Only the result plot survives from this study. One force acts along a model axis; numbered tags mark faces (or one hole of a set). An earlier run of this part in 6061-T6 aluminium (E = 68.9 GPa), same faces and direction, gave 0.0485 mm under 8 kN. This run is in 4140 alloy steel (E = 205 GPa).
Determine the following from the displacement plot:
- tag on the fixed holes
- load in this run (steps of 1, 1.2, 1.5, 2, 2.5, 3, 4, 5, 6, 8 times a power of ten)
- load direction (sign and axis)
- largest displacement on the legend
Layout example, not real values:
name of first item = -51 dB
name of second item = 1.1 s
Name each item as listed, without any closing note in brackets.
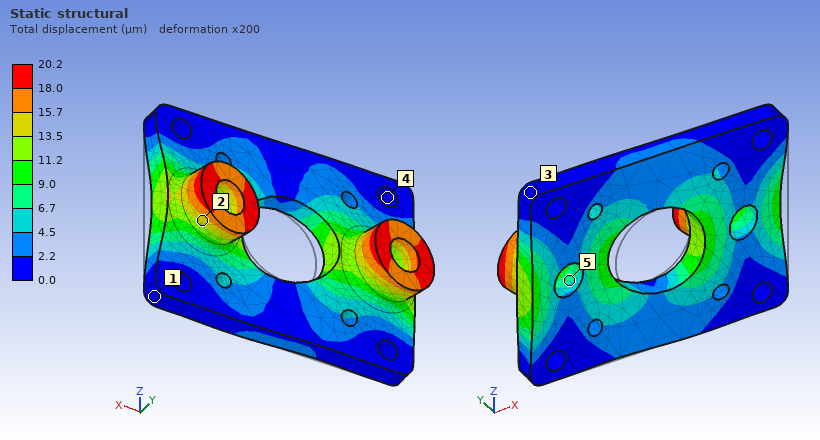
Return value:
tag on the fixed holes = 4
load in this run = 10 kN
load direction = -X
largest displacement on the legend = 20.2 µm
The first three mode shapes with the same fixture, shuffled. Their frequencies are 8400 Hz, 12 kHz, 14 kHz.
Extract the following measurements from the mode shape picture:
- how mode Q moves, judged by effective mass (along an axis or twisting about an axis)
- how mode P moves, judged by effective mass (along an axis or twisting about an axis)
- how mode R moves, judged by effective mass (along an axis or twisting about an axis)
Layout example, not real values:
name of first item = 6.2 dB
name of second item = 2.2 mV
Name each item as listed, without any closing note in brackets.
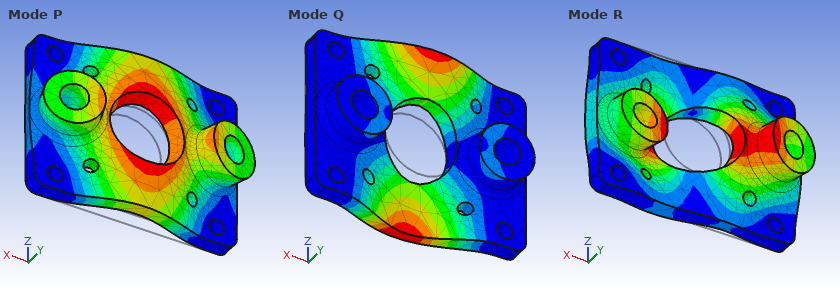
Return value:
how mode Q moves, judged by effective mass = twisting about X
how mode P moves, judged by effective mass = along Y
how mode R moves, judged by effective mass = twisting about Z
